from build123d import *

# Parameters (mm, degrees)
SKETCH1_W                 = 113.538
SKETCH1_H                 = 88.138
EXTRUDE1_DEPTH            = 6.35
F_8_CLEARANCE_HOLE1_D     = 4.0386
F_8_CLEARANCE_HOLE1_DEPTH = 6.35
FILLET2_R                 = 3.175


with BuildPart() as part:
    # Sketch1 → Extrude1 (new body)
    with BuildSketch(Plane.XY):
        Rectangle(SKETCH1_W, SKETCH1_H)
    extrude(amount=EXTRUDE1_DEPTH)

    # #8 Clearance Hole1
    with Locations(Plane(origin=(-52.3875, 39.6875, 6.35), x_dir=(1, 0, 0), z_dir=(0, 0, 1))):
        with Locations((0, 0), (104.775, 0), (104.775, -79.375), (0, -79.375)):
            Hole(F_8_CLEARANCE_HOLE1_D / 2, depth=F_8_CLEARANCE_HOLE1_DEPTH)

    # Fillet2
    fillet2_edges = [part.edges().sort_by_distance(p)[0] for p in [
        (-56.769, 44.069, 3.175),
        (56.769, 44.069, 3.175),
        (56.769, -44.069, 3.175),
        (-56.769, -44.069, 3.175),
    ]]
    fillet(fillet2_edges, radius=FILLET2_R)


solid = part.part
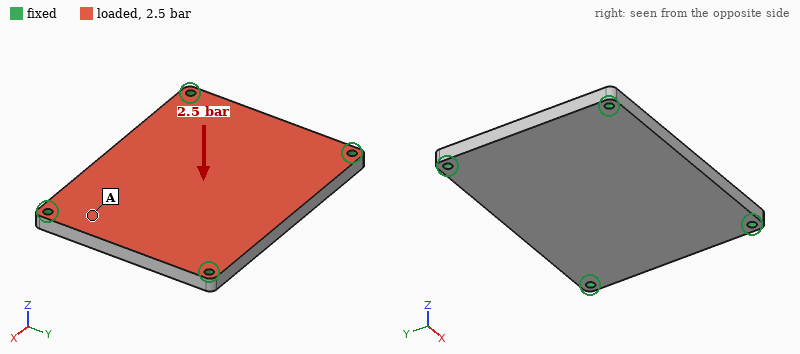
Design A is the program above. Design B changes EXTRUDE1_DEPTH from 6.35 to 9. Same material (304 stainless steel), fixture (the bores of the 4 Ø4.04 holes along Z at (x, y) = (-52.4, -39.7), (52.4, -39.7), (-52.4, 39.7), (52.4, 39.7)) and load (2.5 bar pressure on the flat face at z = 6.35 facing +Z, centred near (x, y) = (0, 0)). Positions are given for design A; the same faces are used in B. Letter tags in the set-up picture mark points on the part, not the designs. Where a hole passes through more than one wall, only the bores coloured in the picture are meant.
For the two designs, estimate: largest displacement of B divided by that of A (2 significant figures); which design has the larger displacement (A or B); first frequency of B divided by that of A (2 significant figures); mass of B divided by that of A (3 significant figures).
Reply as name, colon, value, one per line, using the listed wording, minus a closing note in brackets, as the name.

largest displacement of B divided by that of A: 0.38
which design has the larger displacement: A
first frequency of B divided by that of A: 1.4
mass of B divided by that of A: 1.42
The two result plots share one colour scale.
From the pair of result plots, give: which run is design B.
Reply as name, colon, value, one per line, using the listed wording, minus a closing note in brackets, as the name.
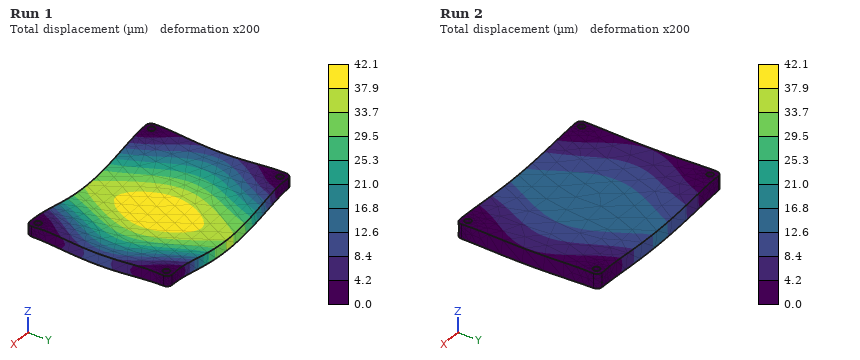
which run is design B: Run 2
